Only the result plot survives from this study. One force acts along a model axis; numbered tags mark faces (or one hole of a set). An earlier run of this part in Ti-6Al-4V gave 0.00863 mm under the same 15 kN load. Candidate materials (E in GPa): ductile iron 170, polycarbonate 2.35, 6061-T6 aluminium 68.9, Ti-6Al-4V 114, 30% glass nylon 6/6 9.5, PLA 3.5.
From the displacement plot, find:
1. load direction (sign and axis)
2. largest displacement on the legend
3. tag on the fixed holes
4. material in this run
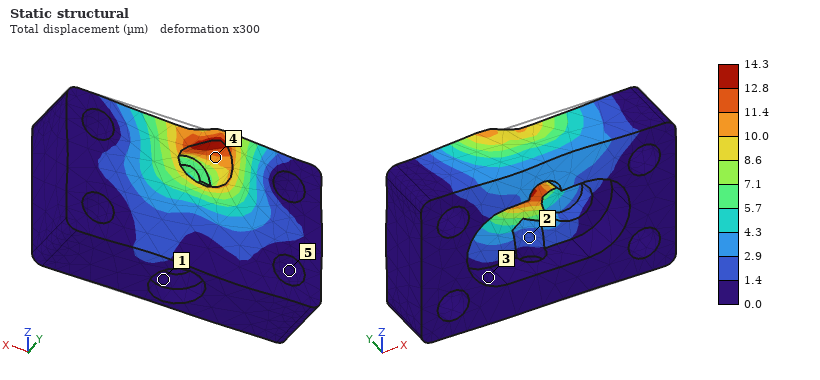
-X
14.3 µm
5
6061-T6 aluminium
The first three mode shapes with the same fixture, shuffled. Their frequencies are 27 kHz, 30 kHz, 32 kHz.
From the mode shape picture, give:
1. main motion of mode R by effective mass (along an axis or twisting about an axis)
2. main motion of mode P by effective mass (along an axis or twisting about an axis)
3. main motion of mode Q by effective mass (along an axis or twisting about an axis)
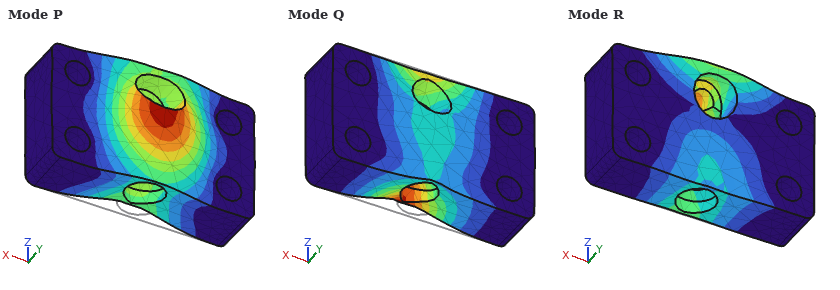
along Z
along Y
along Z
